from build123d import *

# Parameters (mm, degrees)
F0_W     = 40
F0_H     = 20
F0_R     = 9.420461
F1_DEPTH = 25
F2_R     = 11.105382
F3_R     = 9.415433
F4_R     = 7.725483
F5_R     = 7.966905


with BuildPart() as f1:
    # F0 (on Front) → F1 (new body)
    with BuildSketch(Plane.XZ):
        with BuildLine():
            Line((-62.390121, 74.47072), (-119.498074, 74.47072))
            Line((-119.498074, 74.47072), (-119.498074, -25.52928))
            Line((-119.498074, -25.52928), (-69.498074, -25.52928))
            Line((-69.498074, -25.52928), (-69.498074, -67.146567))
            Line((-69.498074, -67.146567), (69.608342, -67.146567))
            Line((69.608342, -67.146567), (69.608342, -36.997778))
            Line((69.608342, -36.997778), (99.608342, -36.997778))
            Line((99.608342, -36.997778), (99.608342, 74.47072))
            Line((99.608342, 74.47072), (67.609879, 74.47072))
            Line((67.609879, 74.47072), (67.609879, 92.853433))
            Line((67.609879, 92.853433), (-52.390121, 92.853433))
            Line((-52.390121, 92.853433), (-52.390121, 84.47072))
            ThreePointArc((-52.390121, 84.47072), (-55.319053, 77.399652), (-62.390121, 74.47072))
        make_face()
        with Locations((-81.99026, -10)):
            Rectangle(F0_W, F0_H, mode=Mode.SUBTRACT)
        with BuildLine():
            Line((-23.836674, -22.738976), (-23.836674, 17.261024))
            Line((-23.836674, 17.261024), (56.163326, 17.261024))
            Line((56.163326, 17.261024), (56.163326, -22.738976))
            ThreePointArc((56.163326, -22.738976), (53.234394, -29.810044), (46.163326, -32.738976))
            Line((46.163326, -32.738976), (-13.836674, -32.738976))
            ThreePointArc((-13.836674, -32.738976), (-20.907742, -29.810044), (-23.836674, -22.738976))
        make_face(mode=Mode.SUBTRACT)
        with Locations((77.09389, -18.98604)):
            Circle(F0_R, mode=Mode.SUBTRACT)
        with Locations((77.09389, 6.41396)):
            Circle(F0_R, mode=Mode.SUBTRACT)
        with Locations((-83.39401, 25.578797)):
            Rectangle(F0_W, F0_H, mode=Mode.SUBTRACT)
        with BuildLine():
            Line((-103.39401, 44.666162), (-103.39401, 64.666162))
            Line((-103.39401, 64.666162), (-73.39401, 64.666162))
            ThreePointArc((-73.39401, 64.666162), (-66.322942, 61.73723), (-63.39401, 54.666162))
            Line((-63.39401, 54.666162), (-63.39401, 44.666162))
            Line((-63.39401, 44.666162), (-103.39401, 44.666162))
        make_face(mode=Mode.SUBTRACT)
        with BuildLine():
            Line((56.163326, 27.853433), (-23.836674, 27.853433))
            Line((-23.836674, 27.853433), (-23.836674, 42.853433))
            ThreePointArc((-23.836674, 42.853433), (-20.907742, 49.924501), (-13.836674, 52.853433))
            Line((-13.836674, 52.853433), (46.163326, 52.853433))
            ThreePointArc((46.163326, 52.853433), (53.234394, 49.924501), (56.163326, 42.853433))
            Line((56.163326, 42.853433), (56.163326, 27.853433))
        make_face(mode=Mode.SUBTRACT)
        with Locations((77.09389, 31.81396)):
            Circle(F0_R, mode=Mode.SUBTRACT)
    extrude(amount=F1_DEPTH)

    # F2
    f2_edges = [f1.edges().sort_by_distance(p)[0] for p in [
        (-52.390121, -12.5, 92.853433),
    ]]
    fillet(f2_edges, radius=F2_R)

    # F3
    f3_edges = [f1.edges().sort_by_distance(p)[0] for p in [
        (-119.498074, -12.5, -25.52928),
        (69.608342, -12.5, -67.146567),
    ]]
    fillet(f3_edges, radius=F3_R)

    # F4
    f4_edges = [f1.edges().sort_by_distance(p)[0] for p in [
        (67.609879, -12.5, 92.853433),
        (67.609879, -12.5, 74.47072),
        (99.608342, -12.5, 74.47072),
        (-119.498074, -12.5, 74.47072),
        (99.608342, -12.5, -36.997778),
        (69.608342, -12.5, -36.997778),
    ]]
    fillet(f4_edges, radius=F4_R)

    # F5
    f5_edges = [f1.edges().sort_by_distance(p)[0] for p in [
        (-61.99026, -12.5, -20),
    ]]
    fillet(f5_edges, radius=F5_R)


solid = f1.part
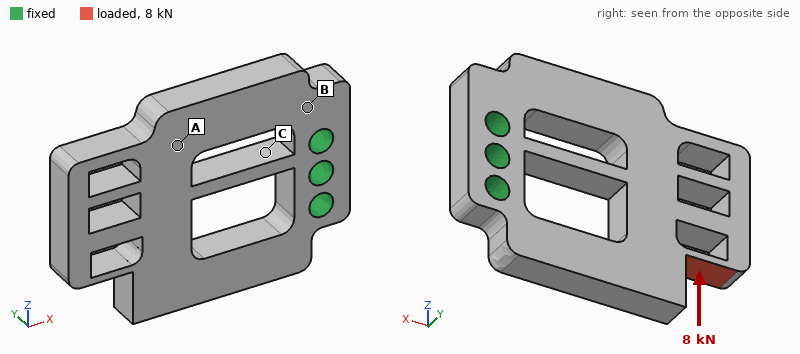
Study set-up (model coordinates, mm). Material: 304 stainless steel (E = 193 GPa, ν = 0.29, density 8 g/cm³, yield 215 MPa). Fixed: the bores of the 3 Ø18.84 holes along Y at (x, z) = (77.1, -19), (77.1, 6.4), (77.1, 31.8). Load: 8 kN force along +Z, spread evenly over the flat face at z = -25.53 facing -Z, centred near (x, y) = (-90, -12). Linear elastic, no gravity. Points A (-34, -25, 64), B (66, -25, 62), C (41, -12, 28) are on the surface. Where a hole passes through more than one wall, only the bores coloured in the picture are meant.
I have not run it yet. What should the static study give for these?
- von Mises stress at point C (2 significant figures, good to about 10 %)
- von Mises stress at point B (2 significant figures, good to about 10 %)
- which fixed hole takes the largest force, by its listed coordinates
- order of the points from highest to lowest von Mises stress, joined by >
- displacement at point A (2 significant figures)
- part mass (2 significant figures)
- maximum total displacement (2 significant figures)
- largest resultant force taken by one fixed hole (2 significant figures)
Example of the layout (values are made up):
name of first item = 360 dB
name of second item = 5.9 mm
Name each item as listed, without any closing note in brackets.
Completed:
von Mises stress at point C = 40 MPa
von Mises stress at point B = 19 MPa
which fixed hole takes the largest force, by its listed coordinates = (77.1, 31.8)
order of the points from highest to lowest von Mises stress, joined by > = C > B > A
displacement at point A = 0.092 mm
part mass = 4.2 kg
maximum total displacement = 0.15 mm
largest resultant force taken by one fixed hole = 15 kN
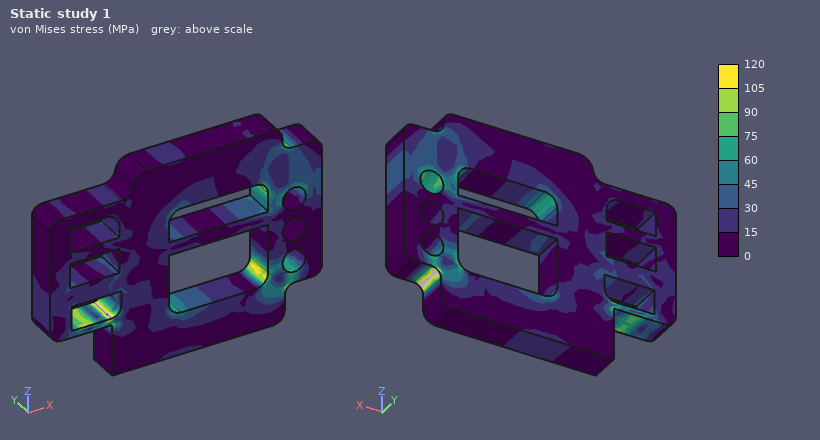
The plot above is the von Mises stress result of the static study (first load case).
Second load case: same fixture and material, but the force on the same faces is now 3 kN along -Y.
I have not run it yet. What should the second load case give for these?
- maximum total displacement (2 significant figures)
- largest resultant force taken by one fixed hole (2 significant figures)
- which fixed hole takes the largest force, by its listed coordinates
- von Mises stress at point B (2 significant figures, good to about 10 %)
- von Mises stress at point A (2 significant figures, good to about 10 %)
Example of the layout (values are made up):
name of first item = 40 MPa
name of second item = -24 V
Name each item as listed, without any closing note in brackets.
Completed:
maximum total displacement = 0.38 mm
largest resultant force taken by one fixed hole = 1.4 kN
which fixed hole takes the largest force, by its listed coordinates = (77.1, -19)
von Mises stress at point B = 44 MPa
von Mises stress at point A = 24 MPa
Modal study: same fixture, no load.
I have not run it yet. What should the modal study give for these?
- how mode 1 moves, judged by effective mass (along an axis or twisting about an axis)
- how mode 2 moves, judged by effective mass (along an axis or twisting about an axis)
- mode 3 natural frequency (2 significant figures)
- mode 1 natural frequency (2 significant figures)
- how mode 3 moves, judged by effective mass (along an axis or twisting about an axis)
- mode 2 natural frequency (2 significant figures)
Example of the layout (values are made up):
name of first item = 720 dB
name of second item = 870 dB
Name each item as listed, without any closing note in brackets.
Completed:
how mode 1 moves, judged by effective mass = along Y
how mode 2 moves, judged by effective mass = along Z
mode 3 natural frequency = 1200 Hz
mode 1 natural frequency = 460 Hz
how mode 3 moves, judged by effective mass = twisting about X
mode 2 natural frequency = 930 Hz
